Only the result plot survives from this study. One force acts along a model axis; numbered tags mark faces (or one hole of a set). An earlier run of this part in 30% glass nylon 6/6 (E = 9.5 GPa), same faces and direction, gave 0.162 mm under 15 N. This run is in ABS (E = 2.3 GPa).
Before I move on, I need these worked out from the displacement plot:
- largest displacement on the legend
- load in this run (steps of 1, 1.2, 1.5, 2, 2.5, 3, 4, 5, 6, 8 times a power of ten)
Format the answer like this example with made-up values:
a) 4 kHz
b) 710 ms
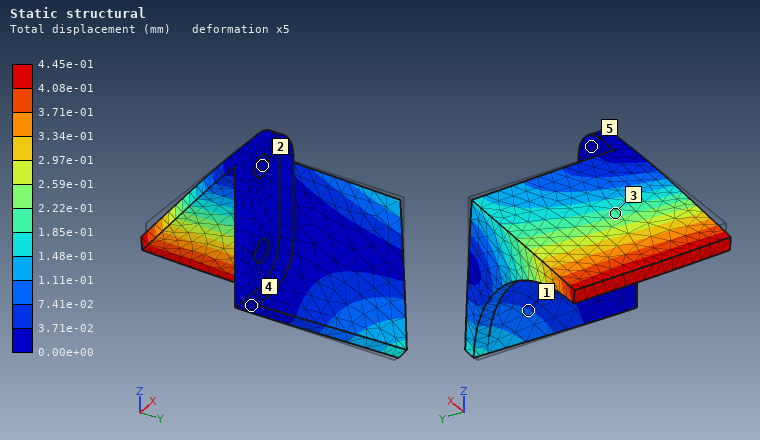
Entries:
a) 4.45e-01 mm
b) 10 N
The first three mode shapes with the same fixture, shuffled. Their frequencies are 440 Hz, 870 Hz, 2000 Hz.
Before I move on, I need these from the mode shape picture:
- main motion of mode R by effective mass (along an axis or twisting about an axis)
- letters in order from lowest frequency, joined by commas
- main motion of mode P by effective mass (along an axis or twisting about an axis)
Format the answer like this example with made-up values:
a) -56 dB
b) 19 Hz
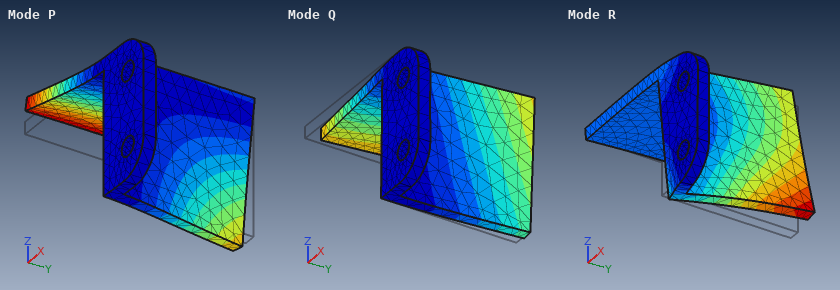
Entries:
a) along Z
b) Q, P, R
c) along Z
